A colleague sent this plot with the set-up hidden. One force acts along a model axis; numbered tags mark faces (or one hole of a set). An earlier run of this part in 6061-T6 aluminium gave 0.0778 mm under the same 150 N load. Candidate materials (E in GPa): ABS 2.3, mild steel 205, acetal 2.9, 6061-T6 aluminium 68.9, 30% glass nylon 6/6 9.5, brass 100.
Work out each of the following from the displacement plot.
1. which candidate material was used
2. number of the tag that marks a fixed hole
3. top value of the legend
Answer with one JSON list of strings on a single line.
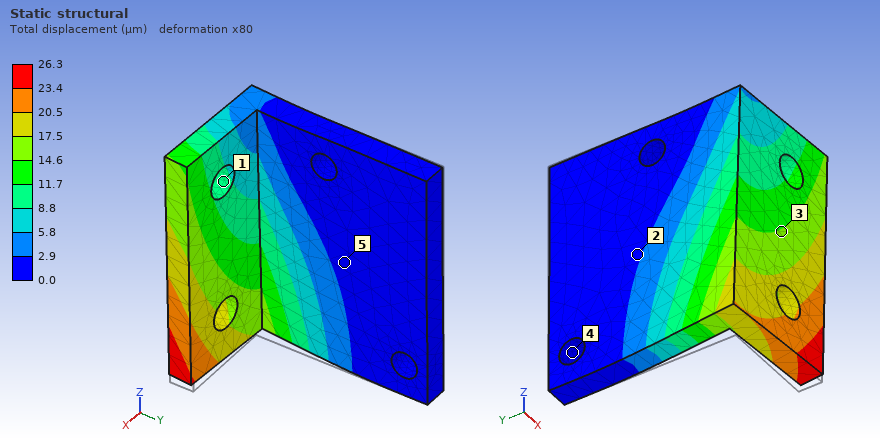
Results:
["mild steel", "4", "26.3 µm"]
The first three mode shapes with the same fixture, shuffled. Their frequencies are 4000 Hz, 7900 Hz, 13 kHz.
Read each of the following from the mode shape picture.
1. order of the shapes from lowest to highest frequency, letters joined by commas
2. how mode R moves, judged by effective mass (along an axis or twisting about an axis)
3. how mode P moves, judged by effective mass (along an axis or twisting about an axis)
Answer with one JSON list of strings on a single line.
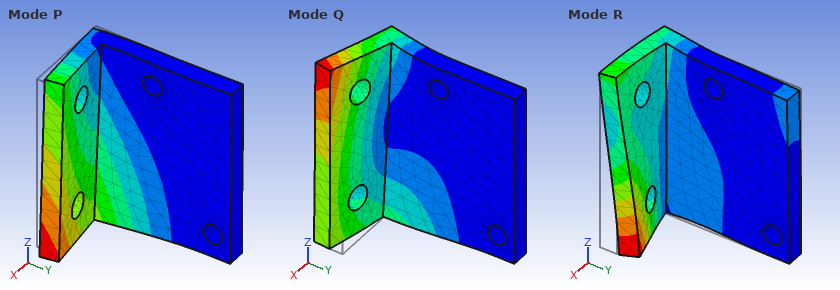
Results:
["P, Q, R", "along X", "along X"]
